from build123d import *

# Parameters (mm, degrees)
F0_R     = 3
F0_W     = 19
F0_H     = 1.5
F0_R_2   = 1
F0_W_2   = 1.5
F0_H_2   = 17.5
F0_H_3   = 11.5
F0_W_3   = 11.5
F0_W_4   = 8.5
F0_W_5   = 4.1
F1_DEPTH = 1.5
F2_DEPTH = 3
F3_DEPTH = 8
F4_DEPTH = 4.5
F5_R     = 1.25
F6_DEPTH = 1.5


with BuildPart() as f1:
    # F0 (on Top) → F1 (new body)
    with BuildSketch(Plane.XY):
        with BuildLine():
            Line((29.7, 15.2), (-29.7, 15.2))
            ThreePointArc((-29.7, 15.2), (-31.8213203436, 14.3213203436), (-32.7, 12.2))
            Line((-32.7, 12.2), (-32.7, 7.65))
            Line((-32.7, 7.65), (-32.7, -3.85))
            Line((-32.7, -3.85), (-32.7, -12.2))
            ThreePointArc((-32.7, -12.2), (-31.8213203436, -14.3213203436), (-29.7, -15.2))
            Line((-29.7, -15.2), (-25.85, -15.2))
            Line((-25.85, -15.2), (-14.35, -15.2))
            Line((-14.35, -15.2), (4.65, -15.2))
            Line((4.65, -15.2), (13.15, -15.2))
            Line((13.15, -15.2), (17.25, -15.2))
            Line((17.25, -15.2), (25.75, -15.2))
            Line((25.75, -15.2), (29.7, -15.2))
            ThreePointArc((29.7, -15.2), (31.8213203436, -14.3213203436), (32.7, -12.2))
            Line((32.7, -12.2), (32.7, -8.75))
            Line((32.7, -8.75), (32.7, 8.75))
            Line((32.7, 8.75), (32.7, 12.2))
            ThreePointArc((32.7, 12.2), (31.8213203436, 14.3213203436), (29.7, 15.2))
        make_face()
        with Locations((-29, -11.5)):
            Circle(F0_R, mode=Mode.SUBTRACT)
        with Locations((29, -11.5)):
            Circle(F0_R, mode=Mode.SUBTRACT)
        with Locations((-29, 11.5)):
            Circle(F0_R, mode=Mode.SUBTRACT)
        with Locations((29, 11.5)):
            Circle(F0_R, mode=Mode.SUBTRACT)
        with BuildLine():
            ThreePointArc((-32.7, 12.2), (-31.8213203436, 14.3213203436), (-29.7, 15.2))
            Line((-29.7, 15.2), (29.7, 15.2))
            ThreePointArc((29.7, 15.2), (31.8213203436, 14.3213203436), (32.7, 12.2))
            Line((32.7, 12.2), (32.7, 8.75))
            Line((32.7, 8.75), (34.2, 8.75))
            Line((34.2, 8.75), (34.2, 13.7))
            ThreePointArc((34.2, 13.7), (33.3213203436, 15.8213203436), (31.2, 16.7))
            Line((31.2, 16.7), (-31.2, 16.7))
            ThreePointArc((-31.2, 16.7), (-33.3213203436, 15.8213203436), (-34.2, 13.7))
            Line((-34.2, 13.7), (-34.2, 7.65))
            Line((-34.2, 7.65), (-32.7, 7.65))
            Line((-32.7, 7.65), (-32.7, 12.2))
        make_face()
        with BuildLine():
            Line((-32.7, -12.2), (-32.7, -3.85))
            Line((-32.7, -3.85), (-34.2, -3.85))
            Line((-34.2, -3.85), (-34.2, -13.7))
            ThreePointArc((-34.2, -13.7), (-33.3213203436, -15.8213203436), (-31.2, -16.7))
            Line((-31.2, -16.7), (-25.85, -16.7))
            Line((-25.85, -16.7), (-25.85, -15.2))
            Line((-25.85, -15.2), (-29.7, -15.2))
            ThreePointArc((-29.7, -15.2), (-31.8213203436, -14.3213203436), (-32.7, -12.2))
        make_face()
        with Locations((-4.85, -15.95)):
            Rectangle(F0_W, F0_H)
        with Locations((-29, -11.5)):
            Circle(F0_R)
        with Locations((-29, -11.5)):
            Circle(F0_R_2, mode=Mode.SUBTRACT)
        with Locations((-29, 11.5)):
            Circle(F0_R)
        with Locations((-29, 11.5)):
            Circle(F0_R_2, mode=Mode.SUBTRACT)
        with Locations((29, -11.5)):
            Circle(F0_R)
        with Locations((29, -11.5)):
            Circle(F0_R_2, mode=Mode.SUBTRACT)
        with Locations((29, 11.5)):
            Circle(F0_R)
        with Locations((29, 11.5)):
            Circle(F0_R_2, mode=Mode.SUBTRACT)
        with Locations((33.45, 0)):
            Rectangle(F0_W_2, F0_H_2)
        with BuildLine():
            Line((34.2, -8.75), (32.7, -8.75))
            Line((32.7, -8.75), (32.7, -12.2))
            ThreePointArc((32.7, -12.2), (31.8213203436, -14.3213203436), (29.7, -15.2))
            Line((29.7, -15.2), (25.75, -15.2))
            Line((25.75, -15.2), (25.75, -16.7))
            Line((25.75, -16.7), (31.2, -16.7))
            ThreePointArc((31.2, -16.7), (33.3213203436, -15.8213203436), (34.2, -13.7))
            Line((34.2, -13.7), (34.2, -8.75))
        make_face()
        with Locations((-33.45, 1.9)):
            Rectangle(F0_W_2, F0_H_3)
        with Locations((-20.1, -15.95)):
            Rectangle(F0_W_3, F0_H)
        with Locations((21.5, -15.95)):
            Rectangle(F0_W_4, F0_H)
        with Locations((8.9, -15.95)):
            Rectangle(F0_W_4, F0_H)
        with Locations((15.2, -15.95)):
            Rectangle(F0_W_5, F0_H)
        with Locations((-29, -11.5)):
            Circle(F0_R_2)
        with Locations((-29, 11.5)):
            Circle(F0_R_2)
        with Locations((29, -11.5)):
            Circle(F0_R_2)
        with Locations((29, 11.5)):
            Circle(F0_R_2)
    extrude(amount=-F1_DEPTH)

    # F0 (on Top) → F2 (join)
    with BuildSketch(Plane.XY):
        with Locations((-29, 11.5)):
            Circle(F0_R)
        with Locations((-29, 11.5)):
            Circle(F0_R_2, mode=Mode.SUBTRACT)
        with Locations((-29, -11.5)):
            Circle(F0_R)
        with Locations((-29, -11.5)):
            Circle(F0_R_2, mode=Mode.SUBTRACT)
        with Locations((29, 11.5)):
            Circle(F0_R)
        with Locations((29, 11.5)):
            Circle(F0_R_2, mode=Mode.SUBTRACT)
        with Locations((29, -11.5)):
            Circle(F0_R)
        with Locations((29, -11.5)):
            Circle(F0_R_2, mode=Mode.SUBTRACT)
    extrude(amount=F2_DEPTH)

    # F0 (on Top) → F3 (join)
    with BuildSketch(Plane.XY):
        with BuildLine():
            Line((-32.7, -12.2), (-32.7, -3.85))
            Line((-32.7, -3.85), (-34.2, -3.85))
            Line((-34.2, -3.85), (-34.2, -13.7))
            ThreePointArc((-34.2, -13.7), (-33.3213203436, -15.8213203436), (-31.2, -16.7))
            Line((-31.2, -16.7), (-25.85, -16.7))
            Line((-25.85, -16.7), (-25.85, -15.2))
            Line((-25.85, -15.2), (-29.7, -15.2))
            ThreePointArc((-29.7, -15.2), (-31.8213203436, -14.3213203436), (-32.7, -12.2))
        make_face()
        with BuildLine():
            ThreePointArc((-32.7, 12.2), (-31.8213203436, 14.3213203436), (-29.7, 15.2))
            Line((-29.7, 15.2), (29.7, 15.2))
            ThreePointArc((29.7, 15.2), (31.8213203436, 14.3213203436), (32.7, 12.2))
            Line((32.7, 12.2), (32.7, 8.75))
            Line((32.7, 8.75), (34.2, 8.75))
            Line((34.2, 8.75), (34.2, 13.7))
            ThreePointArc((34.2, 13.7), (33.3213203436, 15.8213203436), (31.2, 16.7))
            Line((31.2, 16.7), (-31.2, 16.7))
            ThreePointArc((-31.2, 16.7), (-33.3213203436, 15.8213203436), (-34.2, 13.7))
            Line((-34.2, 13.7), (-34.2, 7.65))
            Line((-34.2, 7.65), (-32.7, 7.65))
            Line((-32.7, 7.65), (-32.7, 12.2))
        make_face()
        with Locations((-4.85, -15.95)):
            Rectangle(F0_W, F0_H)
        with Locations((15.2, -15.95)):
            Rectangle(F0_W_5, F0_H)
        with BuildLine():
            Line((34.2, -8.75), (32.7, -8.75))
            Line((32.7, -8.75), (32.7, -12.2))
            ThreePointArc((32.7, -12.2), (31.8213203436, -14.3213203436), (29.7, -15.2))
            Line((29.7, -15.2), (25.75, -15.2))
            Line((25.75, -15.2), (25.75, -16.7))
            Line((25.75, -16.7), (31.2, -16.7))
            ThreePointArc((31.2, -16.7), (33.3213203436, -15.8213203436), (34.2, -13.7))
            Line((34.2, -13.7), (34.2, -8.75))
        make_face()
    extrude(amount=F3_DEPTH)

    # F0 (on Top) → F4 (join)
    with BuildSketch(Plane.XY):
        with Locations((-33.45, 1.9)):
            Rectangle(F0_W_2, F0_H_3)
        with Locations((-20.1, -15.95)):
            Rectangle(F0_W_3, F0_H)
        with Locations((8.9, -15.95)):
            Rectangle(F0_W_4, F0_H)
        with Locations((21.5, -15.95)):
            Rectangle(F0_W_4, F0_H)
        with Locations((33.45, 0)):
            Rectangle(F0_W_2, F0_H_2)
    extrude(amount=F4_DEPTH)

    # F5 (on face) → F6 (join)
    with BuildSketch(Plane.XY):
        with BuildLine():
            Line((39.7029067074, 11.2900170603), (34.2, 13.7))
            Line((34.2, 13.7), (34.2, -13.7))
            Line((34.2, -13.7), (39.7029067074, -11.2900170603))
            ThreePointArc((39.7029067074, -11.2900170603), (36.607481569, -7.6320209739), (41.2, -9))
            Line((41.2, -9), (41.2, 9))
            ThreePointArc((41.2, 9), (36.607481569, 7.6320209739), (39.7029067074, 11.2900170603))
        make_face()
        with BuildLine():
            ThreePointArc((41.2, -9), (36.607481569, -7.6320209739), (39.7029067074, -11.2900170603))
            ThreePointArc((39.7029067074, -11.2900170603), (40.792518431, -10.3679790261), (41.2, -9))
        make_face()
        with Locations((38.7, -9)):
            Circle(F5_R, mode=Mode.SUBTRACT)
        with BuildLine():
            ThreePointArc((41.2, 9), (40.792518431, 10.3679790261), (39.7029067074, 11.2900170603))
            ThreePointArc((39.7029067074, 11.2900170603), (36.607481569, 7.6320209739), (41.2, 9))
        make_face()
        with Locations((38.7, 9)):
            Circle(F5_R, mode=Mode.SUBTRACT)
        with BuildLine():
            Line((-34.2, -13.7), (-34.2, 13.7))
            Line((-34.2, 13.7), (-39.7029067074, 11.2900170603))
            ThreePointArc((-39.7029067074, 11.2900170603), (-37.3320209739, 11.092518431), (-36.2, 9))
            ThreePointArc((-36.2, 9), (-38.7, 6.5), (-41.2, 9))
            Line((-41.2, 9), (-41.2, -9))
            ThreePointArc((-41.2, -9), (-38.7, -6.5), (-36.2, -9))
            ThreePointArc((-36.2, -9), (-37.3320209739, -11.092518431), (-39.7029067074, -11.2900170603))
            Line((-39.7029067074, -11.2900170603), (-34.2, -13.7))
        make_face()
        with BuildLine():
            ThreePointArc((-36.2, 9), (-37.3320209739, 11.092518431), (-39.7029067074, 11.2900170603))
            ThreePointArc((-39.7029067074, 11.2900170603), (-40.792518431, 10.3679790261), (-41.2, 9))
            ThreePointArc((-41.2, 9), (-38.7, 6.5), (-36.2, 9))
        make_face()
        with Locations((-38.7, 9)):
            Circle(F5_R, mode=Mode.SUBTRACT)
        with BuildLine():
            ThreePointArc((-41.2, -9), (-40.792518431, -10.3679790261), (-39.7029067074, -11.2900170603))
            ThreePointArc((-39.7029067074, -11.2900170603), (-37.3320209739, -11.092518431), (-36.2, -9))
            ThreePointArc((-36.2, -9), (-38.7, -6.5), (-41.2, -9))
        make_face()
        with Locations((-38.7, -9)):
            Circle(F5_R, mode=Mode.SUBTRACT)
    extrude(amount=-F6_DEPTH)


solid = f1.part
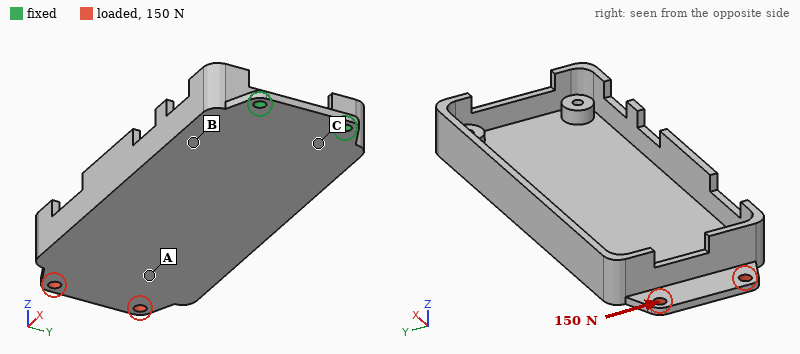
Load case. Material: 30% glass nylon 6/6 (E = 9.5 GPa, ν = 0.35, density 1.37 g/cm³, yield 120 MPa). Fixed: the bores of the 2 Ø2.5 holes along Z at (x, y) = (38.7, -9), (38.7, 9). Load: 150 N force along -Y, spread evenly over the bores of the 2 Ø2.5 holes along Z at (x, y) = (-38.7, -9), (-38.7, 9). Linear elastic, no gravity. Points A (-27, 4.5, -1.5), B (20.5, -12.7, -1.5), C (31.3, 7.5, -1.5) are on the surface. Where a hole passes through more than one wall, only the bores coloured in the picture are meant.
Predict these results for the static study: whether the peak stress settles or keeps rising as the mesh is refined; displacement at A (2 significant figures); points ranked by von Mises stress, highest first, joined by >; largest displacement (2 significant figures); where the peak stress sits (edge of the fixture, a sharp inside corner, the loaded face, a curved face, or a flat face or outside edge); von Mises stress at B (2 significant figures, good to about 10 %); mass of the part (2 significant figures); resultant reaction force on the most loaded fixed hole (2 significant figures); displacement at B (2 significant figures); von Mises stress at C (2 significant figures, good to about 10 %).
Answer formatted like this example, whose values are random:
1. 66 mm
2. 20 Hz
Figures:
1. keeps rising
2. 0.63 mm
3. C > B > A
4. 0.81 mm
5. edge of the fixture
6. 23 MPa
7. 8.6 g
8. 620 N
9. 0.19 mm
10. 37 MPa
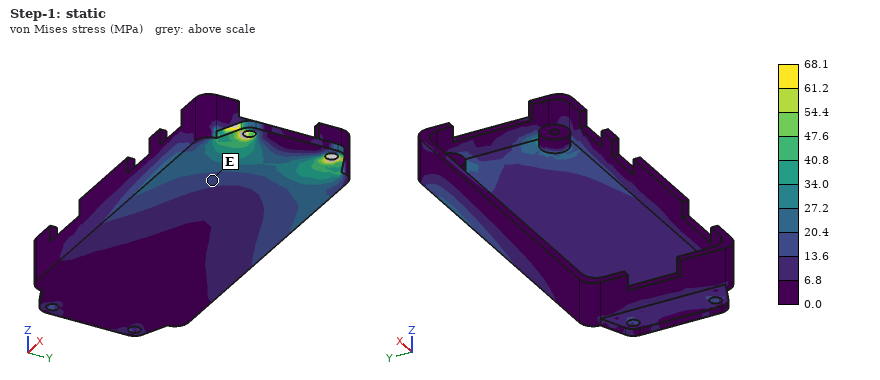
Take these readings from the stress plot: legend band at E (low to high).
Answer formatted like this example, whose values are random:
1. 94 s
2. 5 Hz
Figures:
1. 13.6 to 20.4 MPa
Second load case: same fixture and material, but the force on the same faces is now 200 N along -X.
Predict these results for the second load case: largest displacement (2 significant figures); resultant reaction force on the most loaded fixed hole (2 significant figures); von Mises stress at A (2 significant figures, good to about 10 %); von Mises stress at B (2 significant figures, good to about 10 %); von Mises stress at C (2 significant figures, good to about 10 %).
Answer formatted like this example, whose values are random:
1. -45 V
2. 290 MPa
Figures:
1. 0.22 mm
2. 100 N
3. 4.5 MPa
4. 4.3 MPa
5. 6.1 MPa
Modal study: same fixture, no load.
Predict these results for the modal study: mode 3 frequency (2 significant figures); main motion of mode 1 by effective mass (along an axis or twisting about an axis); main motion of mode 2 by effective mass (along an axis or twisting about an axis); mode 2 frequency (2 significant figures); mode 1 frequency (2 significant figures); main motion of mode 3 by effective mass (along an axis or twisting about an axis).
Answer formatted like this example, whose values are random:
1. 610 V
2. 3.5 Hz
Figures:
1. 1300 Hz
2. along Z
3. twisting about X
4. 460 Hz
5. 130 Hz
6. along Y
